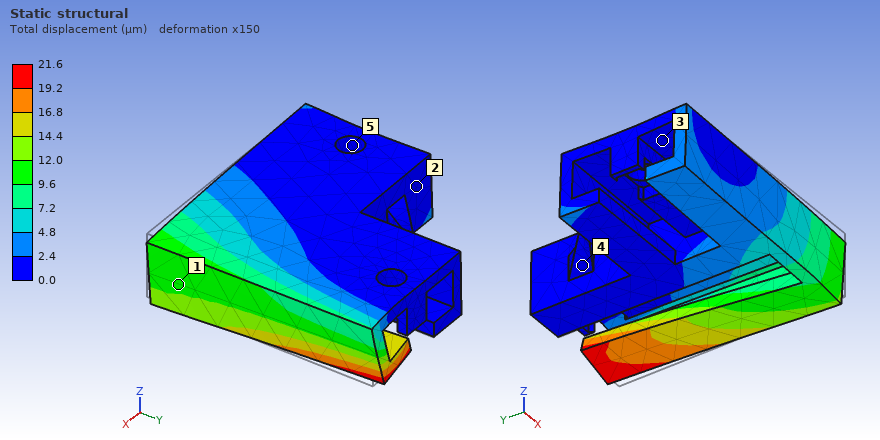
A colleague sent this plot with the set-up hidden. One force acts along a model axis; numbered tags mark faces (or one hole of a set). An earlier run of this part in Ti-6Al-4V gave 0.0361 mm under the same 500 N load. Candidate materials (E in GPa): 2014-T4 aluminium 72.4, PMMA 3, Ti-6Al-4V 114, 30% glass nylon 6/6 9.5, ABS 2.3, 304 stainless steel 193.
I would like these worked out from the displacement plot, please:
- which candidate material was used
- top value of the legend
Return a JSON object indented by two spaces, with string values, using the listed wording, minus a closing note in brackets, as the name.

{
  "which candidate material was used": "304 stainless steel",
  "top value of the legend": "21.6 µm"
}
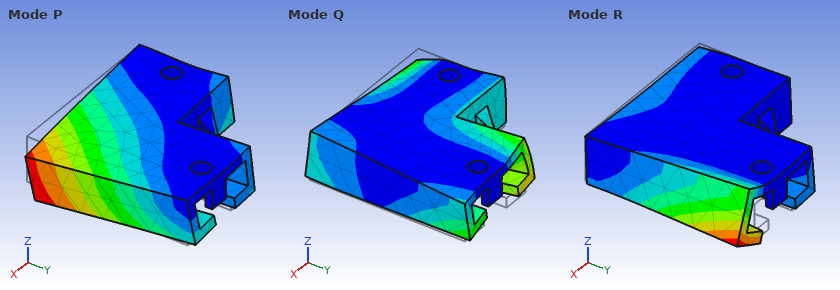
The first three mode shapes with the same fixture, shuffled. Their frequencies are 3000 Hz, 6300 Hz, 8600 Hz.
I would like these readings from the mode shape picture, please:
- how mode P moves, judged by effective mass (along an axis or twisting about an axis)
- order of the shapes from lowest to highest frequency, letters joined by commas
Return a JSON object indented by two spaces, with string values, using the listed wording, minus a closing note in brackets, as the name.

{
  "how mode P moves, judged by effective mass": "along Z",
  "order of the shapes from lowest to highest frequency, letters joined by commas": "P, R, Q"
}
